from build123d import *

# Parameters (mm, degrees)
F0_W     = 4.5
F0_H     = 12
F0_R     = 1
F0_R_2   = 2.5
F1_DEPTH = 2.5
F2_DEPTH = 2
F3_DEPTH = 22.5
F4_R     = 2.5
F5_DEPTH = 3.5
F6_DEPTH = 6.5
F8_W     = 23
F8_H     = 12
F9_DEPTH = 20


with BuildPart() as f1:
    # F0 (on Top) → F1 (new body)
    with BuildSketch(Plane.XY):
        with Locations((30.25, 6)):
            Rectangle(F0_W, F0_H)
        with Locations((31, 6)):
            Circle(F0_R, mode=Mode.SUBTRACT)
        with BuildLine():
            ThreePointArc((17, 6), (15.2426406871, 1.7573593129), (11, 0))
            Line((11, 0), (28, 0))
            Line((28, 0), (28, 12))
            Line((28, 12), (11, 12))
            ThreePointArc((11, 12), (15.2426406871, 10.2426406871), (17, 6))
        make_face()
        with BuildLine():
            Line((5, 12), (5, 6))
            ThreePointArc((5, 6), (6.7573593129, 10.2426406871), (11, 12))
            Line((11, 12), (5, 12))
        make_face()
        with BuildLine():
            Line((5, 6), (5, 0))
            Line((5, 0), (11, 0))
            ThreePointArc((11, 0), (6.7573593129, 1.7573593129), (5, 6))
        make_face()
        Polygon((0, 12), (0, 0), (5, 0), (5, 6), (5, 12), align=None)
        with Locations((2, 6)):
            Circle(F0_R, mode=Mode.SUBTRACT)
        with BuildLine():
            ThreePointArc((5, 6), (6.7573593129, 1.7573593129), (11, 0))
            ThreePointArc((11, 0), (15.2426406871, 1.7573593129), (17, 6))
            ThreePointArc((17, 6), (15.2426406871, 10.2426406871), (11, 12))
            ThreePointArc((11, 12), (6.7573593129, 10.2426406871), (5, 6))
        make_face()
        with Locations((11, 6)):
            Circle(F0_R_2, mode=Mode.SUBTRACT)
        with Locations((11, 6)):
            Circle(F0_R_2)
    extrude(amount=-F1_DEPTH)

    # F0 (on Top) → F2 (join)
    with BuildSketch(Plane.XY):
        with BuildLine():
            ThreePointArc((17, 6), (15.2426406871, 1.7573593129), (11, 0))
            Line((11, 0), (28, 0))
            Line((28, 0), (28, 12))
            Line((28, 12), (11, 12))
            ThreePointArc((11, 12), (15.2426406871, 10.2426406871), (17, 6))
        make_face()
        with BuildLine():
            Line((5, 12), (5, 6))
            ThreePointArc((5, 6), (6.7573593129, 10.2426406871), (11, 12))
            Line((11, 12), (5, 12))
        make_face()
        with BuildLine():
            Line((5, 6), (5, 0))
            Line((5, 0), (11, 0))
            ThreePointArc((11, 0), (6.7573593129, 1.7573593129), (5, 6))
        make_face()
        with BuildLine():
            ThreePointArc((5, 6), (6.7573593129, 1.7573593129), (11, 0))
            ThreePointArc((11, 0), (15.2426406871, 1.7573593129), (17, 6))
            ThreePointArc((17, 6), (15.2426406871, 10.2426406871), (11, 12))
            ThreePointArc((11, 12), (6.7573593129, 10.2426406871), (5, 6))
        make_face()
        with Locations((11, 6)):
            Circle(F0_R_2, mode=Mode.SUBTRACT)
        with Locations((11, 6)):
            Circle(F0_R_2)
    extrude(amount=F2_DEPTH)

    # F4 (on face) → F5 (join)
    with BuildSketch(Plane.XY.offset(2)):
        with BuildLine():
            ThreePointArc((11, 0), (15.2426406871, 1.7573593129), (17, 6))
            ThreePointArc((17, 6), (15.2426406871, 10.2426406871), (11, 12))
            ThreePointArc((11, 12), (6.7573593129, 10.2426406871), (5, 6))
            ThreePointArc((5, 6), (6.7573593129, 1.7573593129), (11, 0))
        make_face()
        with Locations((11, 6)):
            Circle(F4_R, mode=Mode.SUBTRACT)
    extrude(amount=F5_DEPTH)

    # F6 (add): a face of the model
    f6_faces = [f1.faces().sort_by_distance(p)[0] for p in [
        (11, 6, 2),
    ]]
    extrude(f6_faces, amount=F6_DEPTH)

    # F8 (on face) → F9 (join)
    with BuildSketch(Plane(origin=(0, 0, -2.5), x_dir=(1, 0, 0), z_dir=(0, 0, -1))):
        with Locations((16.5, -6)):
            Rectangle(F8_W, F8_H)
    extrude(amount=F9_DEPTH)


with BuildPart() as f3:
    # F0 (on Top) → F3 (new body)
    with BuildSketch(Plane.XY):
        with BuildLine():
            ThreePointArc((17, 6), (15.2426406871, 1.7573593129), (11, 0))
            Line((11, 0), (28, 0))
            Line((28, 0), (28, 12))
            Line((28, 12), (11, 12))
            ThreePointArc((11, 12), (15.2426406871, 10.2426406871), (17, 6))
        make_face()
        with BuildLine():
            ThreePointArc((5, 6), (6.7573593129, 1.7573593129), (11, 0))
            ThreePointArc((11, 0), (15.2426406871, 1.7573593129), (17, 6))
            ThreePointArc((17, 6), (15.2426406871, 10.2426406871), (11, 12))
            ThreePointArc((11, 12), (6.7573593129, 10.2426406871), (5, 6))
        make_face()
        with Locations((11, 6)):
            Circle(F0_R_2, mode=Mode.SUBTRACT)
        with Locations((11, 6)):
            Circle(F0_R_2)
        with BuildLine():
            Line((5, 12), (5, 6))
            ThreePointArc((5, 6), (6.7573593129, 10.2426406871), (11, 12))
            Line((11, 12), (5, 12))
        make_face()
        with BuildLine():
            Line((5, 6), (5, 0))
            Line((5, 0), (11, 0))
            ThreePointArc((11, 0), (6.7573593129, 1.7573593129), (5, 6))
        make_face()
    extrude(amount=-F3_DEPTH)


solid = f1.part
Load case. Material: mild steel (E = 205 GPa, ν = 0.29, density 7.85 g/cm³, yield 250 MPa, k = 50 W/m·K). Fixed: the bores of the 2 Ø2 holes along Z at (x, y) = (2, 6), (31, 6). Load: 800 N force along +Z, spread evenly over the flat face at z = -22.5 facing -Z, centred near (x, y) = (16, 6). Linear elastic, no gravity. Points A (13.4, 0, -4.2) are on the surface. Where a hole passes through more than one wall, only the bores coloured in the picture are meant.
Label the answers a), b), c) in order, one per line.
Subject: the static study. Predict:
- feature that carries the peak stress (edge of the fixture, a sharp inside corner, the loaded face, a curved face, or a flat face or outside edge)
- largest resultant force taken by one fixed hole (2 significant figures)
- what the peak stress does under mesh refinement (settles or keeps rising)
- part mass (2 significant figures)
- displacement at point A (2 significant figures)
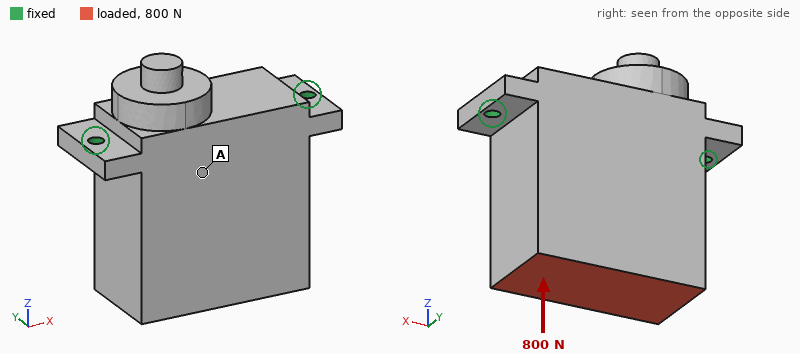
a) edge of the fixture
b) 400 N
c) keeps rising
d) 59 g
e) 2.2 µm
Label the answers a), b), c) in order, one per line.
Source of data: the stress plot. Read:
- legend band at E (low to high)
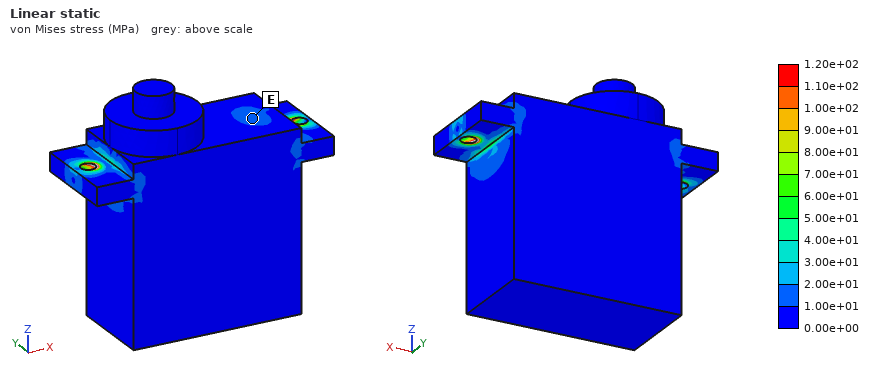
a) 1.00e+01 to 2.00e+01 MPa
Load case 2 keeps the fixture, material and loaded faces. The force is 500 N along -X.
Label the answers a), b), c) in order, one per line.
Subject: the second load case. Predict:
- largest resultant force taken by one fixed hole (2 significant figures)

a) 480 N
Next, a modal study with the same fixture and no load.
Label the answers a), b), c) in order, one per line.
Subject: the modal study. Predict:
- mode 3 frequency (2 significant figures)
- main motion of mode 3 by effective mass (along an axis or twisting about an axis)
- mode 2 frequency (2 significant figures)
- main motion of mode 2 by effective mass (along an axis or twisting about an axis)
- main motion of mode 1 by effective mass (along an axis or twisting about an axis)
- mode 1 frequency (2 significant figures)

a) 13 kHz
b) along Z
c) 12 kHz
d) along X
e) along Y
f) 2800 Hz
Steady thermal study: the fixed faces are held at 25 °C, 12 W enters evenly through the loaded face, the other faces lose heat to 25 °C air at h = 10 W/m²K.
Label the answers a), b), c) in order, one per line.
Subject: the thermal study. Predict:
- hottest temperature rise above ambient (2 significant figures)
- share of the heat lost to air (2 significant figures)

a) 40 K
b) 5.2 %
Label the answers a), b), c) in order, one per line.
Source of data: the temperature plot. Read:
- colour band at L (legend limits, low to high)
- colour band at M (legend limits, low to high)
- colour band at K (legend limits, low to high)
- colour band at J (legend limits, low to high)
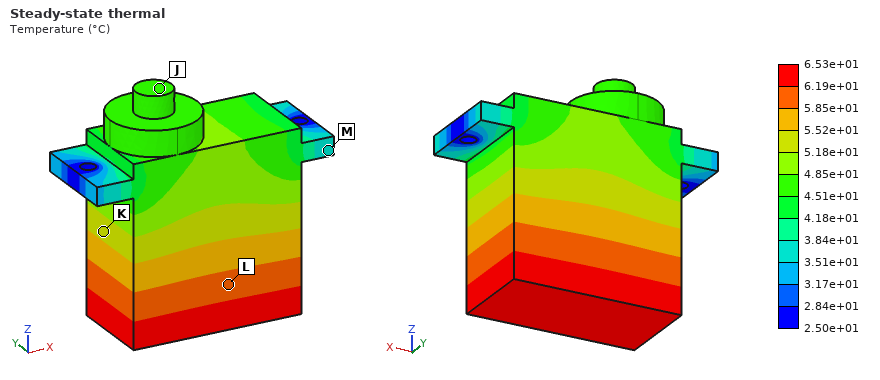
a) 5.85e+01 to 6.19e+01 °C
b) 3.51e+01 to 3.84e+01 °C
c) 5.18e+01 to 5.52e+01 °C
d) 4.51e+01 to 4.85e+01 °C
